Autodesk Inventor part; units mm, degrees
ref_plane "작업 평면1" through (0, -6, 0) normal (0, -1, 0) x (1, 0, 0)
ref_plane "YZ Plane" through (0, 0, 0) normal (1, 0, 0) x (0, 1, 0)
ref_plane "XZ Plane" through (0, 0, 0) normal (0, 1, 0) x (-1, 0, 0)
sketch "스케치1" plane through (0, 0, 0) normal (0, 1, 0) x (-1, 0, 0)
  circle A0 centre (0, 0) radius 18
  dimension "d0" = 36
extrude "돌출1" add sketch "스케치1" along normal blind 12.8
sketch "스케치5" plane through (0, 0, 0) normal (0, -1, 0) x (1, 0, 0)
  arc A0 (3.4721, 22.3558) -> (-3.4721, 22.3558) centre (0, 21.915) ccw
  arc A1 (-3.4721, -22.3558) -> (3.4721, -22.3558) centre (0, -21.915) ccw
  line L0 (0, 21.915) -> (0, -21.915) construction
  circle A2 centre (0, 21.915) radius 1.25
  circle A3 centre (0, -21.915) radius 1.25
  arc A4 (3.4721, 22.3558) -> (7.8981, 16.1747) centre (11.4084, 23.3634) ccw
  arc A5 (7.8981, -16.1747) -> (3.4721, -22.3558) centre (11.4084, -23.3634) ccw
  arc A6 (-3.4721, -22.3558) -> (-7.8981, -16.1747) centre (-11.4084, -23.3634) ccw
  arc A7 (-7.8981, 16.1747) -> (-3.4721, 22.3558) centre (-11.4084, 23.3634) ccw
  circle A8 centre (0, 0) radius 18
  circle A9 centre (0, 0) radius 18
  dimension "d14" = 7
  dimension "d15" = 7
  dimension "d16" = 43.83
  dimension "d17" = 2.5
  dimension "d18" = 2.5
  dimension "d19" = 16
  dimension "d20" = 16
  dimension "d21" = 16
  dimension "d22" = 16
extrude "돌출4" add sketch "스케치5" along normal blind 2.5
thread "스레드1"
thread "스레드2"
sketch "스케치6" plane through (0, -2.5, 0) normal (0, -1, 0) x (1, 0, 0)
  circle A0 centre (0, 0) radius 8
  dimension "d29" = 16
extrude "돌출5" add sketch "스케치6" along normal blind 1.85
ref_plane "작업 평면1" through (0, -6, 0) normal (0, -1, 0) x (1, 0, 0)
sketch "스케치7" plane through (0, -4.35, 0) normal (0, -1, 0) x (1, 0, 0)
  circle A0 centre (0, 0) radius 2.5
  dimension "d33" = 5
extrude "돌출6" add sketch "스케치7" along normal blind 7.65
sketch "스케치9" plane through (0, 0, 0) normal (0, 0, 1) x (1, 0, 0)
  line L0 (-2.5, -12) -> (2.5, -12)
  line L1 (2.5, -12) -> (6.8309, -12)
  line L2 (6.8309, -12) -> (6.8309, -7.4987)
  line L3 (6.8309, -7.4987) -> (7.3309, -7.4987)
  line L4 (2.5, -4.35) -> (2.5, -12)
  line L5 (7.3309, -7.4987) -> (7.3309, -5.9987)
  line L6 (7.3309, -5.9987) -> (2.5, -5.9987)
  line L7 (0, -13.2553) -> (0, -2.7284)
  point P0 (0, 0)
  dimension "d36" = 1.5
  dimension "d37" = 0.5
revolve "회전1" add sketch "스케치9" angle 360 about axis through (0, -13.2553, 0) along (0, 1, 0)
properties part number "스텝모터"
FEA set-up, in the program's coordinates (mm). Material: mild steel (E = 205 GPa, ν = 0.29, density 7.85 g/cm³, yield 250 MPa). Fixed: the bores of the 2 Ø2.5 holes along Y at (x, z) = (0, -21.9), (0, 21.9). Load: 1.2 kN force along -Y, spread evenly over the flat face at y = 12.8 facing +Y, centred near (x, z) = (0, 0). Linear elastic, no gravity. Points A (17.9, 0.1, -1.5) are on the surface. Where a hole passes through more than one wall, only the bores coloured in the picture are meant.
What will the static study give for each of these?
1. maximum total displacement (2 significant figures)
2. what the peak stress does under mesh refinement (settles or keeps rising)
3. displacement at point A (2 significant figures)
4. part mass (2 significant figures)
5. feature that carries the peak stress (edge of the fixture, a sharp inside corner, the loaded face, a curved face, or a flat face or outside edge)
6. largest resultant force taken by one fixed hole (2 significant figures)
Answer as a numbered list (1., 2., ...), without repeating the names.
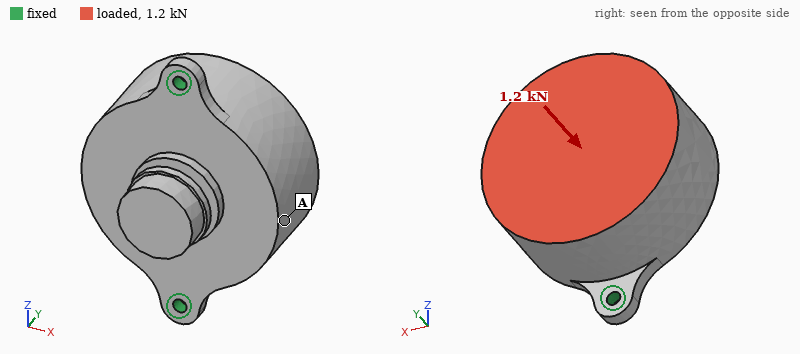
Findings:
1. 5.6 µm
2. keeps rising
3. 5.5 µm
4. 130 g
5. edge of the fixture
6. 680 N
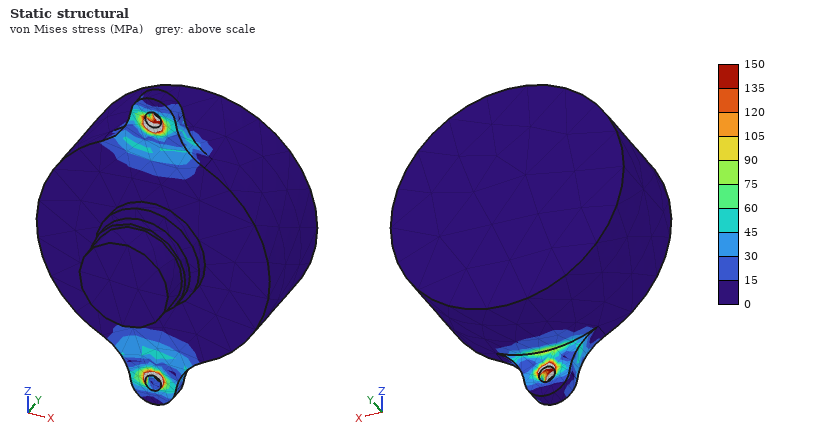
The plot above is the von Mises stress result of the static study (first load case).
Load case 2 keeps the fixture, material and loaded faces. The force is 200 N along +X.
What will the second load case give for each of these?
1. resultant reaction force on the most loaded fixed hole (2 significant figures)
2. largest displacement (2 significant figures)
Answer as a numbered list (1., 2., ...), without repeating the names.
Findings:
1. 100 N
2. 37 µm
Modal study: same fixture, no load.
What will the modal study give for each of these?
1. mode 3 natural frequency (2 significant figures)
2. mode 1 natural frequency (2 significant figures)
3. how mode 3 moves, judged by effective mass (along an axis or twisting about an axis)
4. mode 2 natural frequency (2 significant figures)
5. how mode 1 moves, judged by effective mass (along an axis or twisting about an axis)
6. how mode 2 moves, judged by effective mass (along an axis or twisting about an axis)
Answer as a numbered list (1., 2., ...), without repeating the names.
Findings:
1. 10 kHz
2. 1600 Hz
3. along X
4. 6600 Hz
5. along X
6. along Y
